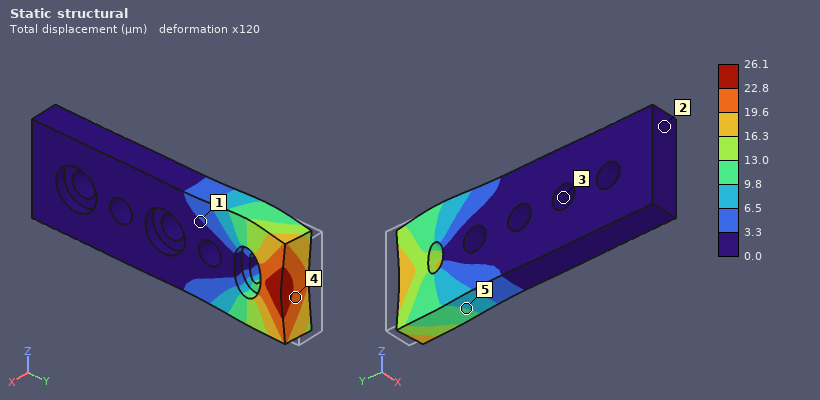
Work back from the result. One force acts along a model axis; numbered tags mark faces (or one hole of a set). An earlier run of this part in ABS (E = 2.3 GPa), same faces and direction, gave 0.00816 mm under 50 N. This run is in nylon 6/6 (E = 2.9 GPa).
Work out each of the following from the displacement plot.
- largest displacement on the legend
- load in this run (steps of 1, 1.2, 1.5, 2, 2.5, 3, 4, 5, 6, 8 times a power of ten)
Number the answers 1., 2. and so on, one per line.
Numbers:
1. 26.1 µm
2. 200 N
